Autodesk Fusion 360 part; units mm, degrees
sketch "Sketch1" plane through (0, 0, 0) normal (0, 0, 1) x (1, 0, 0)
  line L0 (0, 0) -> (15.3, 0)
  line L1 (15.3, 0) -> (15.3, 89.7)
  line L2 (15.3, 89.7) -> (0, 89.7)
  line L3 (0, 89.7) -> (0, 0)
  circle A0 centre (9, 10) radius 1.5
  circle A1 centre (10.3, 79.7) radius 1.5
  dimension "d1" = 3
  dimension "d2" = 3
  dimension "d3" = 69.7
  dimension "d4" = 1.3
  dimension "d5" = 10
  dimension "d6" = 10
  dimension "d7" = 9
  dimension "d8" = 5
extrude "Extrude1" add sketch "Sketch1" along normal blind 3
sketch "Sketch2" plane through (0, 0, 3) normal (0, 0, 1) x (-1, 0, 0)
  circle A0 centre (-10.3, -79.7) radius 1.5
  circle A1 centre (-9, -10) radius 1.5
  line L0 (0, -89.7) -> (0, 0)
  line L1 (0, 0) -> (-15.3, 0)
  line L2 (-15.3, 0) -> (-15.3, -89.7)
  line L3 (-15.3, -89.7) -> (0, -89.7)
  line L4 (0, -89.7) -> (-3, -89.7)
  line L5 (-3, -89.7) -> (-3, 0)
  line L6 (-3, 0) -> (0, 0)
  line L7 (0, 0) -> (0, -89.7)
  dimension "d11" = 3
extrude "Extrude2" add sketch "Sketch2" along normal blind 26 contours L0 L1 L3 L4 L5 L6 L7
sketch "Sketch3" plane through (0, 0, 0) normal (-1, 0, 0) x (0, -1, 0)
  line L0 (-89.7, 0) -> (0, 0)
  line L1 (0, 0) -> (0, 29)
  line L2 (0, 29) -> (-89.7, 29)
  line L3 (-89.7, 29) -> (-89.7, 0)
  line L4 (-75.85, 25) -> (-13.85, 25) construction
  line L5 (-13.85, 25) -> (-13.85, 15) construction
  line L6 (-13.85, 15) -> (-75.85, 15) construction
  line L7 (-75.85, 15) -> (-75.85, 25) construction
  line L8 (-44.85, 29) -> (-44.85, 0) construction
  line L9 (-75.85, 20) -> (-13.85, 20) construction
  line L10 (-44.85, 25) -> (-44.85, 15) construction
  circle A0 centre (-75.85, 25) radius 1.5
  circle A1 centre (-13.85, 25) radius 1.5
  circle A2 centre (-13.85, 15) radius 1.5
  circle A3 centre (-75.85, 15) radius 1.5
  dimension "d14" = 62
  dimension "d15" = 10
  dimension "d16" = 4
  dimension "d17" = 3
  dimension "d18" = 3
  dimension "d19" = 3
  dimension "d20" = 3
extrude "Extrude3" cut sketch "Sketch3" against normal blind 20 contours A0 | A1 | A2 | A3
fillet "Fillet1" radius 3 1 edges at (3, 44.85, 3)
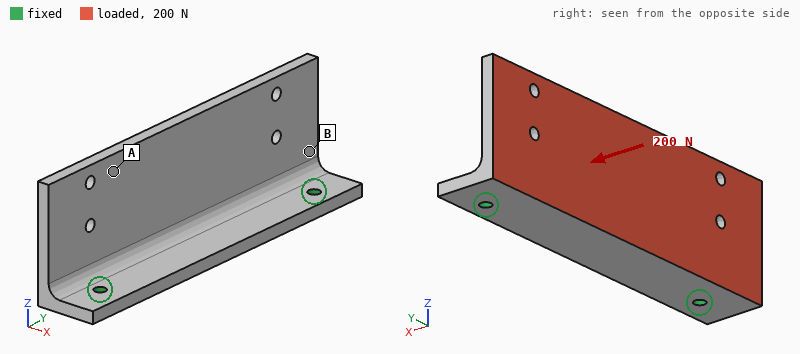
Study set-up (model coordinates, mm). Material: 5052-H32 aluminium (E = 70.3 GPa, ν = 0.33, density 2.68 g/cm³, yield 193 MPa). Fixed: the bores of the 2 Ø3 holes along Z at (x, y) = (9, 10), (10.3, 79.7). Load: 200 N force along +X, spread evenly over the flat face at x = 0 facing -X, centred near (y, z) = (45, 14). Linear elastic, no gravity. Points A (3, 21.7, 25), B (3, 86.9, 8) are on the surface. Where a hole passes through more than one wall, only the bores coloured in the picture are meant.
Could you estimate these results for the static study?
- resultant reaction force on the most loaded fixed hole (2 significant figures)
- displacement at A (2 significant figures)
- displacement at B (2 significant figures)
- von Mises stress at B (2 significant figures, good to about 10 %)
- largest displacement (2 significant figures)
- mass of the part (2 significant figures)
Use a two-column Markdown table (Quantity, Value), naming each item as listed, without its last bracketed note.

| Quantity | Value |
|---|---|
| resultant reaction force on the most loaded fixed hole | 110 N |
| displacement at A | 0.087 mm |
| displacement at B | 0.019 mm |
| von Mises stress at B | 13 MPa |
| largest displacement | 0.12 mm |
| mass of the part | 30 g |
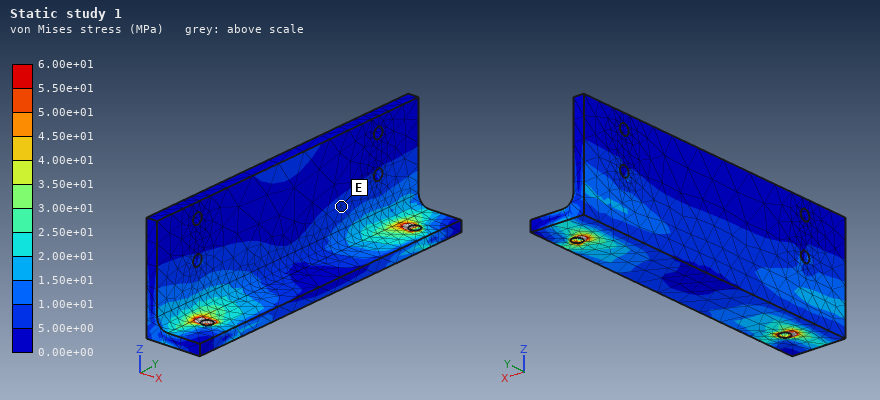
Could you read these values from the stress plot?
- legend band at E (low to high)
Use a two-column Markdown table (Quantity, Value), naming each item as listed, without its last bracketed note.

| Quantity | Value |
|---|---|
| legend band at E | 5.00e+00 to 1.00e+01 MPa |
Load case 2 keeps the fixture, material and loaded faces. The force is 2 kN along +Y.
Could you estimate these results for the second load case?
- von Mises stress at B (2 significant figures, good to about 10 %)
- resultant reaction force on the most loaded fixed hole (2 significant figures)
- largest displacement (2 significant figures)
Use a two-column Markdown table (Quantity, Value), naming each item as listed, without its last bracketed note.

| Quantity | Value |
|---|---|
| von Mises stress at B | 15 MPa |
| resultant reaction force on the most loaded fixed hole | 1.2 kN |
| largest displacement | 52 µm |
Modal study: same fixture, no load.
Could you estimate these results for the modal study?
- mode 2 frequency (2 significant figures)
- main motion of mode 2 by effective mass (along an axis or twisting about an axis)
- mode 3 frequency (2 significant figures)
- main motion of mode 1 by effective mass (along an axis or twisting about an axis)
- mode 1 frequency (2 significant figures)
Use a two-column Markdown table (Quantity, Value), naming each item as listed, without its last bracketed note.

| Quantity | Value |
|---|---|
| mode 2 frequency | 3200 Hz |
| main motion of mode 2 by effective mass | twisting about Z |
| mode 3 frequency | 4900 Hz |
| main motion of mode 1 by effective mass | along X |
| mode 1 frequency | 1800 Hz |
